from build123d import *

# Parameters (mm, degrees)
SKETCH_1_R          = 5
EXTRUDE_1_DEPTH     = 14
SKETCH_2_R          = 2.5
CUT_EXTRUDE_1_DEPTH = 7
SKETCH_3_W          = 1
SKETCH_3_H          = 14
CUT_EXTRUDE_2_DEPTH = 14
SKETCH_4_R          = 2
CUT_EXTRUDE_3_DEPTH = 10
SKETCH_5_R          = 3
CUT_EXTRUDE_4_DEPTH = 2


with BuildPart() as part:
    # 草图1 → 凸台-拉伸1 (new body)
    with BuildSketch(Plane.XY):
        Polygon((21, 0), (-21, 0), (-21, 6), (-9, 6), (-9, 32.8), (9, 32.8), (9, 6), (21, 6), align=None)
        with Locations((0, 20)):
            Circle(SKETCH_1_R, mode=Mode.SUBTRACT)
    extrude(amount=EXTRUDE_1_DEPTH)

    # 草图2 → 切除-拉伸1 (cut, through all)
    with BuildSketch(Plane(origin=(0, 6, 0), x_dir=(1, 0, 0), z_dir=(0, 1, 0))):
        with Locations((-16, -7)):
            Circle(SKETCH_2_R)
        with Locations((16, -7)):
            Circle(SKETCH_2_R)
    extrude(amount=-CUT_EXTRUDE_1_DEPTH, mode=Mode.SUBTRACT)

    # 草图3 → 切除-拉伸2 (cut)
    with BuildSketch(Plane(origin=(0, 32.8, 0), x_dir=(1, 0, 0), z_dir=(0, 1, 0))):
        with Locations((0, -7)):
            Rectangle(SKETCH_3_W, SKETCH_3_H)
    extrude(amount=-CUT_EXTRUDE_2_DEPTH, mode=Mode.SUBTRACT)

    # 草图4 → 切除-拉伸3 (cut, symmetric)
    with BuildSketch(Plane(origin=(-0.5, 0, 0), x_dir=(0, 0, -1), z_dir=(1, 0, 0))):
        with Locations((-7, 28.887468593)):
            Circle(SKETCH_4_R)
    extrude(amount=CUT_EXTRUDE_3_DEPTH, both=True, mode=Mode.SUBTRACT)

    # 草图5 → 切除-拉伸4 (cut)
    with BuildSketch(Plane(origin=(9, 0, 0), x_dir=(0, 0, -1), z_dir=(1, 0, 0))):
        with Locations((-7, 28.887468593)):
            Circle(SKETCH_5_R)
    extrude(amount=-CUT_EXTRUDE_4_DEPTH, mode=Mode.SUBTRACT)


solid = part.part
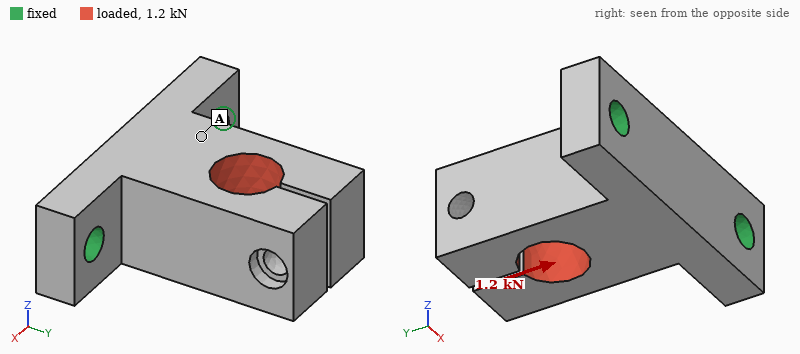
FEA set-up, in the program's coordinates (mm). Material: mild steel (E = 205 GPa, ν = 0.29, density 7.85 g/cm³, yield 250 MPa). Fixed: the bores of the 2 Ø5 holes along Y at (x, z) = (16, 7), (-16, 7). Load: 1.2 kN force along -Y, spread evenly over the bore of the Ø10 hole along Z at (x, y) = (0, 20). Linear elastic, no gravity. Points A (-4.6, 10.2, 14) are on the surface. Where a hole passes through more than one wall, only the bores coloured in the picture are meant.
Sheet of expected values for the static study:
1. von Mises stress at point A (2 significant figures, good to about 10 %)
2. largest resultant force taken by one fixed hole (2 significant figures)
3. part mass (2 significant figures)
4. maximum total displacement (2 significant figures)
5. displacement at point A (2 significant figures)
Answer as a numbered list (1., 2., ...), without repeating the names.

1. 8.8 MPa
2. 640 N
3. 67 g
4. 8.7 µm
5. 1.7 µm
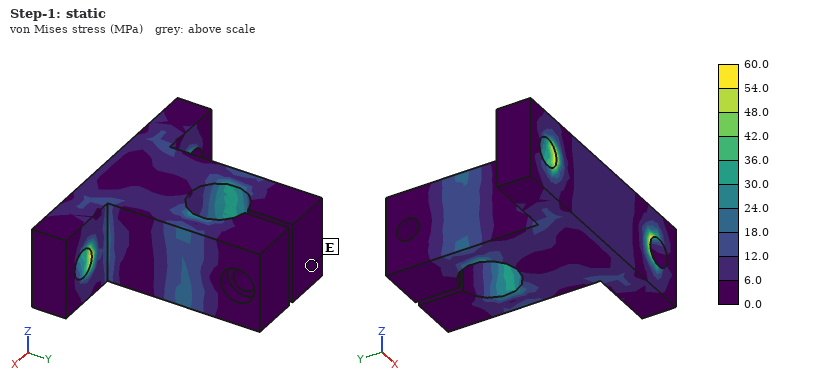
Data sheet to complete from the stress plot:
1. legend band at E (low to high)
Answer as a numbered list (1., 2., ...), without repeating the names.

1. 0.0 to 6.0 MPa
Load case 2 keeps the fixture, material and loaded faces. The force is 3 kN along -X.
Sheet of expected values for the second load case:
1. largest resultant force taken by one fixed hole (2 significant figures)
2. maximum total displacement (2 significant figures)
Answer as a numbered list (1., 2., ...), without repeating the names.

1. 2.6 kN
2. 43 µm
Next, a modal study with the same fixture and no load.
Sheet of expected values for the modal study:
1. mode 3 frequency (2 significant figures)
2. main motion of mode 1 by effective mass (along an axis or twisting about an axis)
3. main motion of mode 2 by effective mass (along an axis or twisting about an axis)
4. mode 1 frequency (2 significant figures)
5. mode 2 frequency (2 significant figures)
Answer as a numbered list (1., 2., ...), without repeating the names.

1. 7700 Hz
2. along Z
3. along X
4. 5200 Hz
5. 6900 Hz
